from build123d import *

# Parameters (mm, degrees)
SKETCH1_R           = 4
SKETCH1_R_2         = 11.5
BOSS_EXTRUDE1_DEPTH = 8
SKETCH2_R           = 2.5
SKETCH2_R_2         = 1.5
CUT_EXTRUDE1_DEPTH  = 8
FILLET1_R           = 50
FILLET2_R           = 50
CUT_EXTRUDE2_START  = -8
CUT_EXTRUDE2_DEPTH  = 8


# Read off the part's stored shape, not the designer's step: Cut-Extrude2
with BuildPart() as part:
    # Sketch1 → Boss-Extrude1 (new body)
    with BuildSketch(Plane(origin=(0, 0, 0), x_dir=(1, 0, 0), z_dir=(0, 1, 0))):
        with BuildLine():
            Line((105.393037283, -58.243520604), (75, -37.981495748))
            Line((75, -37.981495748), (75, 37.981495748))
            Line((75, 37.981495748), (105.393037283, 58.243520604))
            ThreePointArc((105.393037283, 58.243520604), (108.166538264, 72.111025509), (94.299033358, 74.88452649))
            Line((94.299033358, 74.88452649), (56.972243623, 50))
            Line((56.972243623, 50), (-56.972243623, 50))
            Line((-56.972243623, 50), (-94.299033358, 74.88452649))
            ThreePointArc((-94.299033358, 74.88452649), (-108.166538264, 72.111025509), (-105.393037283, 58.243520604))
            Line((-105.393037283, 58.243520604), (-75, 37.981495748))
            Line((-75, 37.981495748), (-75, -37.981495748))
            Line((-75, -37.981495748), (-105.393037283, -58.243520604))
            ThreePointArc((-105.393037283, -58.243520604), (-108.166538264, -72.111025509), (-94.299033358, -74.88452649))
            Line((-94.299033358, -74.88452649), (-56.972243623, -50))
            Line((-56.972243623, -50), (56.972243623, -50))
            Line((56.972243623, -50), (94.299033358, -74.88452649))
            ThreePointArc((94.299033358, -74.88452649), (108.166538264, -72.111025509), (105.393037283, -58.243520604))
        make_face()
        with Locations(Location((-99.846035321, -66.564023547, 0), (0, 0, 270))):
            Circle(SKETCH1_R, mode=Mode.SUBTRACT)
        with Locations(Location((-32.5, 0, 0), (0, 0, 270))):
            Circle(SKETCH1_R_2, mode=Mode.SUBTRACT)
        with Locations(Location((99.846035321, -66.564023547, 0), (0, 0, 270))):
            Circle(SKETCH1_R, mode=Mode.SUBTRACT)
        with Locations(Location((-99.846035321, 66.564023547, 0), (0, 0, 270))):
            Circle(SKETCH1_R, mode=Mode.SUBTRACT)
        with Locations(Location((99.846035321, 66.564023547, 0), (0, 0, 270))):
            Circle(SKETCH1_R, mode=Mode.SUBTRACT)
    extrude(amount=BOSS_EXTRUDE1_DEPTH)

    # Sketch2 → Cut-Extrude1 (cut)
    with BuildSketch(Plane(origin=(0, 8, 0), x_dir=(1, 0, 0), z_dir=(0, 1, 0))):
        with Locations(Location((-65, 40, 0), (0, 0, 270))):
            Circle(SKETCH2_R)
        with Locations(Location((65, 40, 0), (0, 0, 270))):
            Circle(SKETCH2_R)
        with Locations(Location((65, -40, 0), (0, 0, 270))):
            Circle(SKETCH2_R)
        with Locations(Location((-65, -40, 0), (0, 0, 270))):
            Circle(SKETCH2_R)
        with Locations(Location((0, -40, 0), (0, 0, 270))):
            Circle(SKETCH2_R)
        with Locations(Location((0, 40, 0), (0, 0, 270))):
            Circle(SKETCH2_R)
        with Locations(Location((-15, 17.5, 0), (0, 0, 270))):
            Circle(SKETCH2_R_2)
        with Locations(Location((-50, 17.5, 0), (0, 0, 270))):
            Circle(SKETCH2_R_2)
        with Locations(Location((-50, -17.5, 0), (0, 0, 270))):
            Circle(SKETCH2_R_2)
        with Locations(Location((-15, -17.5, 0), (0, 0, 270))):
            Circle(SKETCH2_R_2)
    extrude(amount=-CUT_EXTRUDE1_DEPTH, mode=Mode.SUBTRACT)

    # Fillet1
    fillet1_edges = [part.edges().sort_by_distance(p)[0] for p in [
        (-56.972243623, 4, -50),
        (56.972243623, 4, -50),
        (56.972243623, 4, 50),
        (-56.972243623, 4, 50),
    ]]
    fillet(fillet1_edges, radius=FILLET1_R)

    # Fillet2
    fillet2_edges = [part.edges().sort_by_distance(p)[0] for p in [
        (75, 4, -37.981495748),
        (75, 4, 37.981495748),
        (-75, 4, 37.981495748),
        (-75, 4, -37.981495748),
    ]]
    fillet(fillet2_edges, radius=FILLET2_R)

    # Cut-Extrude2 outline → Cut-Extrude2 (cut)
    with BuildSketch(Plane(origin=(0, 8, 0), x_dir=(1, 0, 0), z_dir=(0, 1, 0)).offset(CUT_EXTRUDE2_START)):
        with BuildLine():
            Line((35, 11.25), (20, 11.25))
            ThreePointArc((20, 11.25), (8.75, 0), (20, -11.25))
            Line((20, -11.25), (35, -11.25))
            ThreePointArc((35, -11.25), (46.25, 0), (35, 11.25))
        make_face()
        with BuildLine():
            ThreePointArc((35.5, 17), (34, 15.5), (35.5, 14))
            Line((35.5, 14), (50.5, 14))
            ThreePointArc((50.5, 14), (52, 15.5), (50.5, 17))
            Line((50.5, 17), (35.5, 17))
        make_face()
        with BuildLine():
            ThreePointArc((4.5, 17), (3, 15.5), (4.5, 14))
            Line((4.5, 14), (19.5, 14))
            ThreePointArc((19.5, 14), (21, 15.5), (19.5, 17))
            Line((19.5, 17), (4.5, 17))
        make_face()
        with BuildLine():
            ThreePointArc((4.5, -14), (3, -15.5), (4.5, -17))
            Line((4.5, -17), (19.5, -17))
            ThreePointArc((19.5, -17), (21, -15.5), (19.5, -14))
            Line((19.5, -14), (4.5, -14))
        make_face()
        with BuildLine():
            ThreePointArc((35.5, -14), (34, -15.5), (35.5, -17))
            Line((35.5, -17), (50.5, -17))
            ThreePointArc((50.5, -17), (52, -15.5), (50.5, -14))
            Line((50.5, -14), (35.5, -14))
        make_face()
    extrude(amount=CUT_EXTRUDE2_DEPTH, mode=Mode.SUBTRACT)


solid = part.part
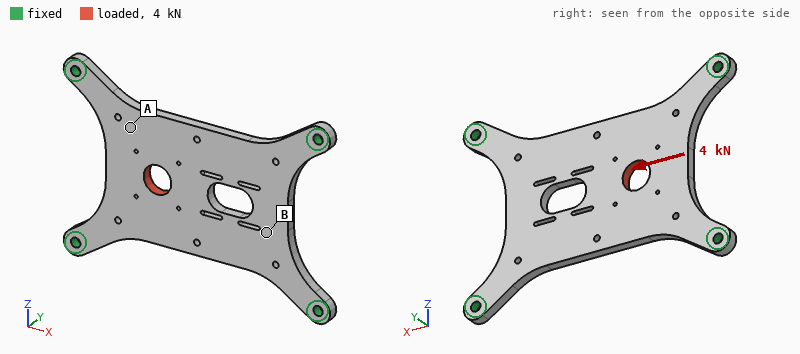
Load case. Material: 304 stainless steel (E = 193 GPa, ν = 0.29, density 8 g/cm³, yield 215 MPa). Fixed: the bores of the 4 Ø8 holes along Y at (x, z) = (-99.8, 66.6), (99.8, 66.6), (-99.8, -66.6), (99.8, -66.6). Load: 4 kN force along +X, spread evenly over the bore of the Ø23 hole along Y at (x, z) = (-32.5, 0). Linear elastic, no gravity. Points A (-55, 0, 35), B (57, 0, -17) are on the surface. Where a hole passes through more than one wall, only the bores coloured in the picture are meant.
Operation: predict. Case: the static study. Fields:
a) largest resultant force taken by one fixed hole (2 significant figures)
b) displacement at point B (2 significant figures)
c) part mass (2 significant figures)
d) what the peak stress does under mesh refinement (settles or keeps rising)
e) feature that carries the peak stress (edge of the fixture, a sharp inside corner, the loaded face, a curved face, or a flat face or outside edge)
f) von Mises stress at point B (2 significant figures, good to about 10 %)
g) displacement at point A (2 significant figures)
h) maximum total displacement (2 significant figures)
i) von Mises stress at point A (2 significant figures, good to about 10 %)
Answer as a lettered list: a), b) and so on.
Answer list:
a) 1.4 kN
b) 2.2 µm
c) 1.1 kg
d) keeps rising
e) edge of the fixture
f) 1.7 MPa
g) 2.7 µm
h) 4.4 µm
i) 4.5 MPa
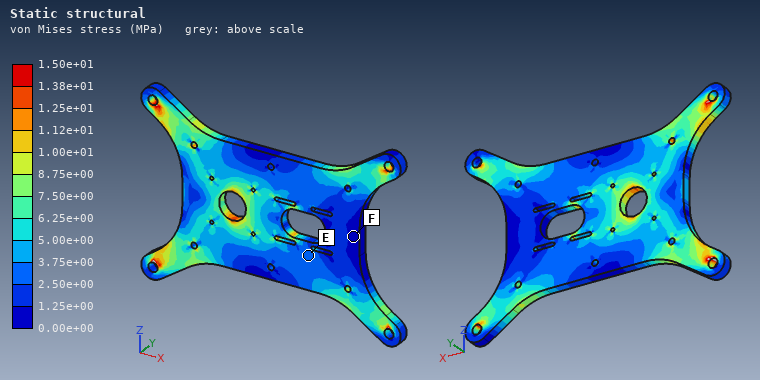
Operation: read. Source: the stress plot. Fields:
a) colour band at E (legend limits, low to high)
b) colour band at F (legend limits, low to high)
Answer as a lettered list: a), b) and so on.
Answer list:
a) 2.50e+00 to 3.75e+00 MPa
b) 0.00e+00 to 1.25e+00 MPa
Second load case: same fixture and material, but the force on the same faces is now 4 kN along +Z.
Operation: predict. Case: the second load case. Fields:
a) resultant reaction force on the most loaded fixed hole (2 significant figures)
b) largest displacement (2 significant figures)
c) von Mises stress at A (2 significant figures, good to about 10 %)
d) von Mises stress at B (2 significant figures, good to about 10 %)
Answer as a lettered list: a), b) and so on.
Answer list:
a) 1.9 kN
b) 6.9 µm
c) 5.5 MPa
d) 2.2 MPa
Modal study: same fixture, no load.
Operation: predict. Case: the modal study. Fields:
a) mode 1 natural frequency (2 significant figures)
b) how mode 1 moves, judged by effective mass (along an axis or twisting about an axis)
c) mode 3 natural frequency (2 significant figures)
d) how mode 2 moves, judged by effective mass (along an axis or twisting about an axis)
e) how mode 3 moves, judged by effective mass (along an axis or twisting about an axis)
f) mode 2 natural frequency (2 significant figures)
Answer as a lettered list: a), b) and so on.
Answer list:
a) 720 Hz
b) along Y
c) 1800 Hz
d) twisting about X
e) twisting about Z
f) 1500 Hz
